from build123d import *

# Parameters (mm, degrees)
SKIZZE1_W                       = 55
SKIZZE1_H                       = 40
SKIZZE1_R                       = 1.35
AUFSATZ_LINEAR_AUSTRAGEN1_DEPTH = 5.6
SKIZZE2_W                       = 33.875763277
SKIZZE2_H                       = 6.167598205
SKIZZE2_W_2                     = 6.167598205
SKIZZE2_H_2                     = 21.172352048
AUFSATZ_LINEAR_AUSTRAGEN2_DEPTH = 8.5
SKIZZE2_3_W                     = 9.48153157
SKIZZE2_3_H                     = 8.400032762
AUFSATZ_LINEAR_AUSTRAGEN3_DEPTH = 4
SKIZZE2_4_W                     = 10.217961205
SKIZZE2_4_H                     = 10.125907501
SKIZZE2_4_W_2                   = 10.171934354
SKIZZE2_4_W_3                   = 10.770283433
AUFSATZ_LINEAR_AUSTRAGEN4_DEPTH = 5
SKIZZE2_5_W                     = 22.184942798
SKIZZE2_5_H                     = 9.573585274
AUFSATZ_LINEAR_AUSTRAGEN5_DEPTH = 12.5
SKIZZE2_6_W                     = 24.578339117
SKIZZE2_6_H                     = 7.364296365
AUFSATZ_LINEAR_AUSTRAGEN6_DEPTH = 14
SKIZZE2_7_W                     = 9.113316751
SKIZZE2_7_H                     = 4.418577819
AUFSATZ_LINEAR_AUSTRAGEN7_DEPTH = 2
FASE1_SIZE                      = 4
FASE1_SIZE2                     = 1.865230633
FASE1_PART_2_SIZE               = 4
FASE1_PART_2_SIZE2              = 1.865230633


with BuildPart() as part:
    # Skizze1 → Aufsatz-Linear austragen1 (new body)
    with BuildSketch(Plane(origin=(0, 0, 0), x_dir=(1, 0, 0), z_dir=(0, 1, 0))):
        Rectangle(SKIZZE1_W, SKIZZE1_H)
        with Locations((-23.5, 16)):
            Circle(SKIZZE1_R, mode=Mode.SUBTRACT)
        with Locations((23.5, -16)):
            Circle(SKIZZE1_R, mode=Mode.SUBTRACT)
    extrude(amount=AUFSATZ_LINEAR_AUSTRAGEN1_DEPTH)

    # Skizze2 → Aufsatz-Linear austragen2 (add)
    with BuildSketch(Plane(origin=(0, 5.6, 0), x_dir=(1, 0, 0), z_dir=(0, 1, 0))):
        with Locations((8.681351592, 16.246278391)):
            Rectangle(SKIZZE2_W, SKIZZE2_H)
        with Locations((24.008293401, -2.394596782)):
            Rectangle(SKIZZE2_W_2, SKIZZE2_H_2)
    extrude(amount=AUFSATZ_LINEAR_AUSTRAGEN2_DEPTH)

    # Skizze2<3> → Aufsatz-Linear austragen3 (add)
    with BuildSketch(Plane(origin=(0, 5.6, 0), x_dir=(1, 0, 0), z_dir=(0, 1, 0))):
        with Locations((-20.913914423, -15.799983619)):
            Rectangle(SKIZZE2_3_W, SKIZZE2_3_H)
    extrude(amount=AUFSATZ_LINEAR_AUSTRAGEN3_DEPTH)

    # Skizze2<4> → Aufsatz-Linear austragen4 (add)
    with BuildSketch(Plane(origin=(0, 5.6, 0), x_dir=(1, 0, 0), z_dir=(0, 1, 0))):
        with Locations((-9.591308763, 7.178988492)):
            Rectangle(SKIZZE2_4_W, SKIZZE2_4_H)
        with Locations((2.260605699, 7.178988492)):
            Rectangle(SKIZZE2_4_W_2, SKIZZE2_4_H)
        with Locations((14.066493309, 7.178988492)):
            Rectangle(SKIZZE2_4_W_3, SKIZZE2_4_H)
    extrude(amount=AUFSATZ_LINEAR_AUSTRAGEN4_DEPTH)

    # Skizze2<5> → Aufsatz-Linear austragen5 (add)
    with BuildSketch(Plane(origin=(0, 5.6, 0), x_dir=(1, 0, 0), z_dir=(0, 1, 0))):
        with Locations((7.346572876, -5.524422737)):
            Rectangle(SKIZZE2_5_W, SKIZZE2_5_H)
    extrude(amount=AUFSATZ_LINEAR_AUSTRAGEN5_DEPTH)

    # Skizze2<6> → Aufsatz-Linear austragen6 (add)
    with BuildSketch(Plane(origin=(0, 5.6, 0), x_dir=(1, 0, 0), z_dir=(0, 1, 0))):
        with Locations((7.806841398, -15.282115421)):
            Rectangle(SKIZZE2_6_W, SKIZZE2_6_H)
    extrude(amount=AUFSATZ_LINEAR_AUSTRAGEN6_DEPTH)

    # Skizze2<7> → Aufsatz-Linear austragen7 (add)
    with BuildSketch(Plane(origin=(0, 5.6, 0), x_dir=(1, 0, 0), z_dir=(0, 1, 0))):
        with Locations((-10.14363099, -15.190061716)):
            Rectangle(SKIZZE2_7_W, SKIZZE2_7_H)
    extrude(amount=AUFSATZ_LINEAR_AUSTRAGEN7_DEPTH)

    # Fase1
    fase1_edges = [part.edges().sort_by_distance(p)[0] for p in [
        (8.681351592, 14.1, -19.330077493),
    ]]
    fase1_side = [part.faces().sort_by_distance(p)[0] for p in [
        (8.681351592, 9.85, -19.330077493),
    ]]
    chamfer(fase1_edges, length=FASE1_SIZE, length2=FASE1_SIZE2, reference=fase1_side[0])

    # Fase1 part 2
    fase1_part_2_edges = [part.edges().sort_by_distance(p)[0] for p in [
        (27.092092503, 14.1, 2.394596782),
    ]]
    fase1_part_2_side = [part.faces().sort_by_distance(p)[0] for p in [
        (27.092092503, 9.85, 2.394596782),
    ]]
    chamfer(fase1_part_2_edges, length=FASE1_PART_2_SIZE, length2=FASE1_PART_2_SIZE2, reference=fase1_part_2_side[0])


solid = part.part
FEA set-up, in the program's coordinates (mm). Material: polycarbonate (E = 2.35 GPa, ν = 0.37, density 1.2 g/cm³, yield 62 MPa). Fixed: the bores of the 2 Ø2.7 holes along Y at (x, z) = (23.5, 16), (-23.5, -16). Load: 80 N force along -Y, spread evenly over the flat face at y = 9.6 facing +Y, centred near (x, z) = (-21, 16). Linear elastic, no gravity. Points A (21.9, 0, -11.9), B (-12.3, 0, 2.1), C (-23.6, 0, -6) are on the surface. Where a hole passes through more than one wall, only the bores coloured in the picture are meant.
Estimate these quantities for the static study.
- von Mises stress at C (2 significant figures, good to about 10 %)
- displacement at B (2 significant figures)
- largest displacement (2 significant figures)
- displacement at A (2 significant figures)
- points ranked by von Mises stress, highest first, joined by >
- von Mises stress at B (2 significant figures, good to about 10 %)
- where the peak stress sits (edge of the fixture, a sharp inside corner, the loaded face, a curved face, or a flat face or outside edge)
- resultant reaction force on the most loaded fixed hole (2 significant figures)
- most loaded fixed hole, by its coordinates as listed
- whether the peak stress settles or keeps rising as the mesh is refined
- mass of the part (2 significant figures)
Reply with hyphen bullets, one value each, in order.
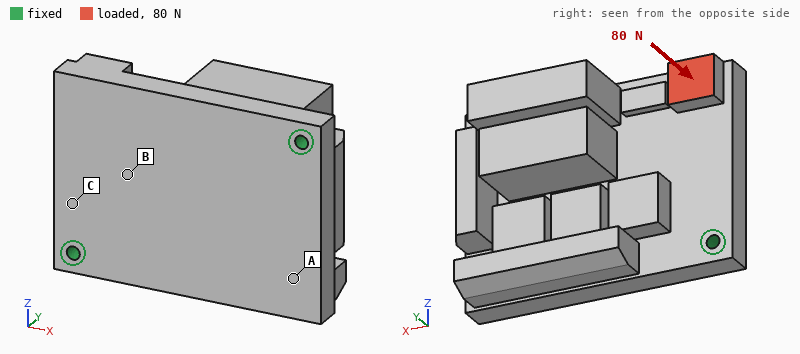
- 7.6 MPa
- 0.22 mm
- 0.81 mm
- 0.24 mm
- C > B > A
- 4.6 MPa
- edge of the fixture
- 55 N
- (-23.5, -16)
- keeps rising
- 27 g
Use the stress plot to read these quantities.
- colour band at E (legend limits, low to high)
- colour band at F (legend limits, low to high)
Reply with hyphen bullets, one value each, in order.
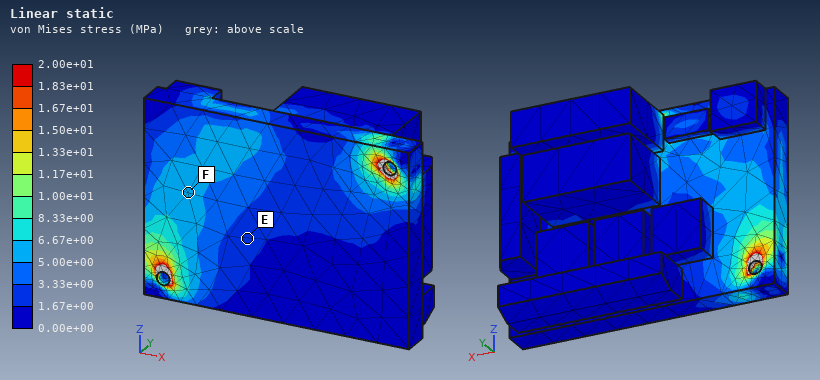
- 1.67e+00 to 3.33e+00 MPa
- 5.00e+00 to 6.67e+00 MPa
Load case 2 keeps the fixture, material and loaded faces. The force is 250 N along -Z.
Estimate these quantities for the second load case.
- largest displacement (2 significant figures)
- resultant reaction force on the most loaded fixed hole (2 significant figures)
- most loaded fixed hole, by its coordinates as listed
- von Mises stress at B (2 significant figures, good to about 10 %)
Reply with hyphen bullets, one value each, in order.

- 0.77 mm
- 220 N
- (-23.5, -16)
- 4.0 MPa
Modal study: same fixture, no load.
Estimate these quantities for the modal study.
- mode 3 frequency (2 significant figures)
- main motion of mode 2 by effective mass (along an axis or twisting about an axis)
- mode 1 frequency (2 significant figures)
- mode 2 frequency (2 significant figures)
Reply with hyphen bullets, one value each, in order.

- 2800 Hz
- along Y
- 810 Hz
- 1300 Hz
